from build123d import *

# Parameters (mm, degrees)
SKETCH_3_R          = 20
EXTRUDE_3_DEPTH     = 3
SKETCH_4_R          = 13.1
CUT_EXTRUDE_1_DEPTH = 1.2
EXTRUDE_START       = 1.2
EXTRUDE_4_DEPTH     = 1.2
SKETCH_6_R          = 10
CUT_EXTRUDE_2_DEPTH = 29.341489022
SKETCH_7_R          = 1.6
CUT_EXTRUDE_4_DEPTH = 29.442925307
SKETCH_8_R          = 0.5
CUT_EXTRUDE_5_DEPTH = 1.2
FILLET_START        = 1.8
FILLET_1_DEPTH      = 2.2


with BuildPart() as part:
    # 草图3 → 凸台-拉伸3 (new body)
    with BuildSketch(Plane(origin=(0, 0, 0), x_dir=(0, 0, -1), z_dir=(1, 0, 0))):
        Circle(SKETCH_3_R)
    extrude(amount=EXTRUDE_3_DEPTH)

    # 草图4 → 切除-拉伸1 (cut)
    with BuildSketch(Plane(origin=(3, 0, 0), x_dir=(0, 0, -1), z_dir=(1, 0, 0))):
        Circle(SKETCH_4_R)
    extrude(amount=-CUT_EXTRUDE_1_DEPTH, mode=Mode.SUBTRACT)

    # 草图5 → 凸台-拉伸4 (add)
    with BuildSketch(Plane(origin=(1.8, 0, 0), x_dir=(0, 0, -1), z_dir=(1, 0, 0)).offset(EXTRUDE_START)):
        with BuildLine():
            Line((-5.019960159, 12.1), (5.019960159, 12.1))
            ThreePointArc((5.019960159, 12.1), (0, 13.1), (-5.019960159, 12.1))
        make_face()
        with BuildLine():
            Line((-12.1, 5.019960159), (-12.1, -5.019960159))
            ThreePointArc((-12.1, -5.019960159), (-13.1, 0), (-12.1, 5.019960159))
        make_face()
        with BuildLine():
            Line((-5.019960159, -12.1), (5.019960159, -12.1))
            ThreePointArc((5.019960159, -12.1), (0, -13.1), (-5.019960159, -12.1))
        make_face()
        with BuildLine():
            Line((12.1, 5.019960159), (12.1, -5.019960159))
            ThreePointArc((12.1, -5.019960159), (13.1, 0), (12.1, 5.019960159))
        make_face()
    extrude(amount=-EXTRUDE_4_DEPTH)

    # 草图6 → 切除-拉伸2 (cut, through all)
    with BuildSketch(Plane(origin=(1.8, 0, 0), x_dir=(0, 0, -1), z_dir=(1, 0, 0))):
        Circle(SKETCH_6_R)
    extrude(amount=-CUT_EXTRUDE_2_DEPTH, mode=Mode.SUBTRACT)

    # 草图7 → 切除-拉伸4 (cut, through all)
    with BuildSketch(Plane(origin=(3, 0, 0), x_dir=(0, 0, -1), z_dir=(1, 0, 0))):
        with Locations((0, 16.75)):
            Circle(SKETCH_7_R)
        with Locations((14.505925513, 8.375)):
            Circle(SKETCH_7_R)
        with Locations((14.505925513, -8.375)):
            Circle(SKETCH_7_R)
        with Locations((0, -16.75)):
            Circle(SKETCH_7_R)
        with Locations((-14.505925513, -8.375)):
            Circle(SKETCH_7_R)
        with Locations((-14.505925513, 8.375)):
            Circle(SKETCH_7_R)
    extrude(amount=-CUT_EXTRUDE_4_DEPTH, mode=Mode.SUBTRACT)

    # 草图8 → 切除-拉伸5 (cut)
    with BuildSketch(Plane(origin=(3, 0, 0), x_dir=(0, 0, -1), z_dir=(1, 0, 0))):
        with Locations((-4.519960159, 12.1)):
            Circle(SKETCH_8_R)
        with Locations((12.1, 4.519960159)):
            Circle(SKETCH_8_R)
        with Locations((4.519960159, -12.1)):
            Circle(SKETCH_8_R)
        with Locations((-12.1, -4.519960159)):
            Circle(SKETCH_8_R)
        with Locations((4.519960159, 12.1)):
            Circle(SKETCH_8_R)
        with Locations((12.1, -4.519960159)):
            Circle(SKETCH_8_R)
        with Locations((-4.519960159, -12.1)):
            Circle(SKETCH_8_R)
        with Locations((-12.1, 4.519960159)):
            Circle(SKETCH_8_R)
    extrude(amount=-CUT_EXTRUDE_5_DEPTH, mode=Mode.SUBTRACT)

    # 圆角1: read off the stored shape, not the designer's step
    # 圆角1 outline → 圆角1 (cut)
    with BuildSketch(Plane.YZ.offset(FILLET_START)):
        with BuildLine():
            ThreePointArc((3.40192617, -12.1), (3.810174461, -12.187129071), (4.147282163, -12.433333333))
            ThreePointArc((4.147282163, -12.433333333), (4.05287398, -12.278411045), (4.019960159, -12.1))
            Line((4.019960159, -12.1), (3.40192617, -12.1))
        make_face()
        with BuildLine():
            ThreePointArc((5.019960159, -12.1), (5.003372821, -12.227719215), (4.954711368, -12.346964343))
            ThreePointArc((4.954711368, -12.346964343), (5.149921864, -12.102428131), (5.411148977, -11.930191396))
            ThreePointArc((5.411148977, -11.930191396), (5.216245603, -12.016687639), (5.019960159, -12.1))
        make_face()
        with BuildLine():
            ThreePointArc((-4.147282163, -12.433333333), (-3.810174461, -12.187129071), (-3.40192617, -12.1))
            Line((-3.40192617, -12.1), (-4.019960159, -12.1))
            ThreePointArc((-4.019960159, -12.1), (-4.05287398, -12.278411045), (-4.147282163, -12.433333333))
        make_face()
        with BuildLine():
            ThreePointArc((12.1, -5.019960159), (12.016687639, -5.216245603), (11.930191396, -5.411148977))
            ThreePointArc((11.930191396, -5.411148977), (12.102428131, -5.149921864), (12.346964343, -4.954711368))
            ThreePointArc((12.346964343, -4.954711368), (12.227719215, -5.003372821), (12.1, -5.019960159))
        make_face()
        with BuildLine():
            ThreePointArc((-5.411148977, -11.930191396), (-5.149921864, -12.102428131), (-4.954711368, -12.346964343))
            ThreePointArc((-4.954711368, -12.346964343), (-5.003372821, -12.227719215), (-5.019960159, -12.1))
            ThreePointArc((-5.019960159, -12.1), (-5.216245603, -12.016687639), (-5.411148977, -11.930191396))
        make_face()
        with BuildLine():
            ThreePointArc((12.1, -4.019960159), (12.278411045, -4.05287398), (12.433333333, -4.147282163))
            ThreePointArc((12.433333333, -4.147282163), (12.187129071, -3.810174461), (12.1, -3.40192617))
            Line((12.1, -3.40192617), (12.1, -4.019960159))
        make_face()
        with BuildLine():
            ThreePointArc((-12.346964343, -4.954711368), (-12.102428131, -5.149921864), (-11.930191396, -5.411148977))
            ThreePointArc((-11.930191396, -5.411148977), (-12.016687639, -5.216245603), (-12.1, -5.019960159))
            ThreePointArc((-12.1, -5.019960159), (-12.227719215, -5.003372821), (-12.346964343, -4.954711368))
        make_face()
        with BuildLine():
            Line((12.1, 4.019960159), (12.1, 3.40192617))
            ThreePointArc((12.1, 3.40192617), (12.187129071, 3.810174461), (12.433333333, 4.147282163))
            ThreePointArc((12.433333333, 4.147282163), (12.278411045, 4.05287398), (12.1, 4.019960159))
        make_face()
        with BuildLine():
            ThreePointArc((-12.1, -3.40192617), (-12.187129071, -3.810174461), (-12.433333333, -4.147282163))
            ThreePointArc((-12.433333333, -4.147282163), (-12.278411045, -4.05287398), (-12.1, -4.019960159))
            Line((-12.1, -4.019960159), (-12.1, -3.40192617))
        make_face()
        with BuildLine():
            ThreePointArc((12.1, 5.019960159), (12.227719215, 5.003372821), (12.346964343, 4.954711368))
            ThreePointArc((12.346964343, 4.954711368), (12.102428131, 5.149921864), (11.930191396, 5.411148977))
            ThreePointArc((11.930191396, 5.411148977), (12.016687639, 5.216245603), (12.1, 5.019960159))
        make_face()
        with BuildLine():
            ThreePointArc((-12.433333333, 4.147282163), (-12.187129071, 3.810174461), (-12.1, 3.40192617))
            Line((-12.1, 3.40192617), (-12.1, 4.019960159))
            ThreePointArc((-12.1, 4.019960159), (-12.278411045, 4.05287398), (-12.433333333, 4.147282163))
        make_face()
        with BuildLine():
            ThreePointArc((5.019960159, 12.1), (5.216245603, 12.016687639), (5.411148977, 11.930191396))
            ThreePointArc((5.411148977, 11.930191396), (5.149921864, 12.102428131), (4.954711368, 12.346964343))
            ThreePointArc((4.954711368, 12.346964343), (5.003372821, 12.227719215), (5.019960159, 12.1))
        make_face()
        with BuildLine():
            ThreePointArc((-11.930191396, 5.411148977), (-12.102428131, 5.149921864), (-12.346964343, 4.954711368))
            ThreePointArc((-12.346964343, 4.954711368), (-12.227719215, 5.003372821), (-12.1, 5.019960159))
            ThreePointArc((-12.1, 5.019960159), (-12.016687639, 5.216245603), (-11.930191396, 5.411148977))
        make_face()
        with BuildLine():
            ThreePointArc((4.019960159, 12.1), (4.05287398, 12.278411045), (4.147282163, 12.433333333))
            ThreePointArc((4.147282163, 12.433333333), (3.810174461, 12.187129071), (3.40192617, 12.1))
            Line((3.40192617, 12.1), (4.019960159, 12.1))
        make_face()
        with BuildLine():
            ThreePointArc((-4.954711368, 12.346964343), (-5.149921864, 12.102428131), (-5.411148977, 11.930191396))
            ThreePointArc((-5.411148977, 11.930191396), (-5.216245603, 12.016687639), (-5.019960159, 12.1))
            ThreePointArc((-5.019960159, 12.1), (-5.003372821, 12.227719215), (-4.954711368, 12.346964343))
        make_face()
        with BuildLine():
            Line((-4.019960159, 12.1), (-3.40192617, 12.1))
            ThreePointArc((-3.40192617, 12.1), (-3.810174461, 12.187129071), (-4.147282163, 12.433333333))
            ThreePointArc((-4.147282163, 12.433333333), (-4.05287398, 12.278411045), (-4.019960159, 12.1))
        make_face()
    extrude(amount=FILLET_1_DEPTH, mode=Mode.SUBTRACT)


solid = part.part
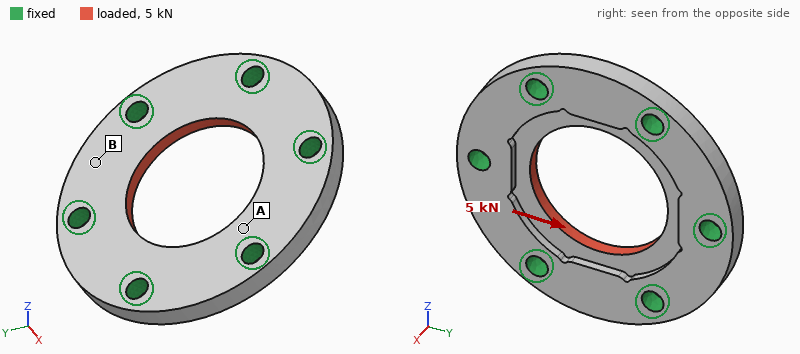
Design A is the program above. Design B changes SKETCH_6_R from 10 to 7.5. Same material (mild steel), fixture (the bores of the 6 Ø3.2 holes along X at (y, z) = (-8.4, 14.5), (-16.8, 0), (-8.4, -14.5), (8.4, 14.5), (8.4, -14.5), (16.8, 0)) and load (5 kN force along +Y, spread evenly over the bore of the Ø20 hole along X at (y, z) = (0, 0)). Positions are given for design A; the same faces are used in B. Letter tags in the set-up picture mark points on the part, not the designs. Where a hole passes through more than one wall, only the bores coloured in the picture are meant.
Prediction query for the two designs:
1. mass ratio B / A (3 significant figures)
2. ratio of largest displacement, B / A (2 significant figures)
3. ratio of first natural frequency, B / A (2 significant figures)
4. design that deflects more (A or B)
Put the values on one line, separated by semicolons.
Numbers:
1.10; 1.3; 0.68; B
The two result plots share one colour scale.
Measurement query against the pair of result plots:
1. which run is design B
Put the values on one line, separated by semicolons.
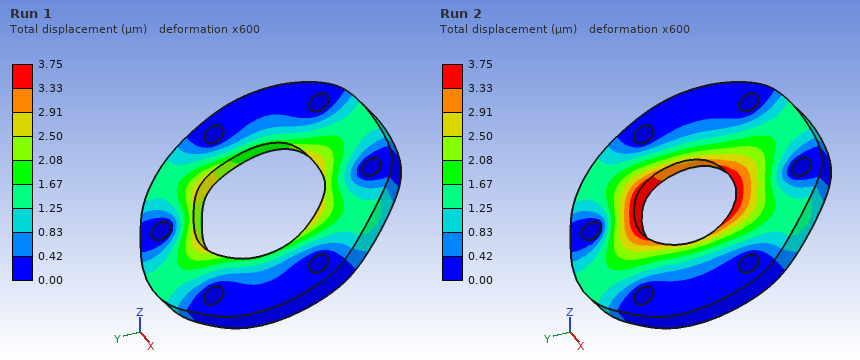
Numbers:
Run 2
